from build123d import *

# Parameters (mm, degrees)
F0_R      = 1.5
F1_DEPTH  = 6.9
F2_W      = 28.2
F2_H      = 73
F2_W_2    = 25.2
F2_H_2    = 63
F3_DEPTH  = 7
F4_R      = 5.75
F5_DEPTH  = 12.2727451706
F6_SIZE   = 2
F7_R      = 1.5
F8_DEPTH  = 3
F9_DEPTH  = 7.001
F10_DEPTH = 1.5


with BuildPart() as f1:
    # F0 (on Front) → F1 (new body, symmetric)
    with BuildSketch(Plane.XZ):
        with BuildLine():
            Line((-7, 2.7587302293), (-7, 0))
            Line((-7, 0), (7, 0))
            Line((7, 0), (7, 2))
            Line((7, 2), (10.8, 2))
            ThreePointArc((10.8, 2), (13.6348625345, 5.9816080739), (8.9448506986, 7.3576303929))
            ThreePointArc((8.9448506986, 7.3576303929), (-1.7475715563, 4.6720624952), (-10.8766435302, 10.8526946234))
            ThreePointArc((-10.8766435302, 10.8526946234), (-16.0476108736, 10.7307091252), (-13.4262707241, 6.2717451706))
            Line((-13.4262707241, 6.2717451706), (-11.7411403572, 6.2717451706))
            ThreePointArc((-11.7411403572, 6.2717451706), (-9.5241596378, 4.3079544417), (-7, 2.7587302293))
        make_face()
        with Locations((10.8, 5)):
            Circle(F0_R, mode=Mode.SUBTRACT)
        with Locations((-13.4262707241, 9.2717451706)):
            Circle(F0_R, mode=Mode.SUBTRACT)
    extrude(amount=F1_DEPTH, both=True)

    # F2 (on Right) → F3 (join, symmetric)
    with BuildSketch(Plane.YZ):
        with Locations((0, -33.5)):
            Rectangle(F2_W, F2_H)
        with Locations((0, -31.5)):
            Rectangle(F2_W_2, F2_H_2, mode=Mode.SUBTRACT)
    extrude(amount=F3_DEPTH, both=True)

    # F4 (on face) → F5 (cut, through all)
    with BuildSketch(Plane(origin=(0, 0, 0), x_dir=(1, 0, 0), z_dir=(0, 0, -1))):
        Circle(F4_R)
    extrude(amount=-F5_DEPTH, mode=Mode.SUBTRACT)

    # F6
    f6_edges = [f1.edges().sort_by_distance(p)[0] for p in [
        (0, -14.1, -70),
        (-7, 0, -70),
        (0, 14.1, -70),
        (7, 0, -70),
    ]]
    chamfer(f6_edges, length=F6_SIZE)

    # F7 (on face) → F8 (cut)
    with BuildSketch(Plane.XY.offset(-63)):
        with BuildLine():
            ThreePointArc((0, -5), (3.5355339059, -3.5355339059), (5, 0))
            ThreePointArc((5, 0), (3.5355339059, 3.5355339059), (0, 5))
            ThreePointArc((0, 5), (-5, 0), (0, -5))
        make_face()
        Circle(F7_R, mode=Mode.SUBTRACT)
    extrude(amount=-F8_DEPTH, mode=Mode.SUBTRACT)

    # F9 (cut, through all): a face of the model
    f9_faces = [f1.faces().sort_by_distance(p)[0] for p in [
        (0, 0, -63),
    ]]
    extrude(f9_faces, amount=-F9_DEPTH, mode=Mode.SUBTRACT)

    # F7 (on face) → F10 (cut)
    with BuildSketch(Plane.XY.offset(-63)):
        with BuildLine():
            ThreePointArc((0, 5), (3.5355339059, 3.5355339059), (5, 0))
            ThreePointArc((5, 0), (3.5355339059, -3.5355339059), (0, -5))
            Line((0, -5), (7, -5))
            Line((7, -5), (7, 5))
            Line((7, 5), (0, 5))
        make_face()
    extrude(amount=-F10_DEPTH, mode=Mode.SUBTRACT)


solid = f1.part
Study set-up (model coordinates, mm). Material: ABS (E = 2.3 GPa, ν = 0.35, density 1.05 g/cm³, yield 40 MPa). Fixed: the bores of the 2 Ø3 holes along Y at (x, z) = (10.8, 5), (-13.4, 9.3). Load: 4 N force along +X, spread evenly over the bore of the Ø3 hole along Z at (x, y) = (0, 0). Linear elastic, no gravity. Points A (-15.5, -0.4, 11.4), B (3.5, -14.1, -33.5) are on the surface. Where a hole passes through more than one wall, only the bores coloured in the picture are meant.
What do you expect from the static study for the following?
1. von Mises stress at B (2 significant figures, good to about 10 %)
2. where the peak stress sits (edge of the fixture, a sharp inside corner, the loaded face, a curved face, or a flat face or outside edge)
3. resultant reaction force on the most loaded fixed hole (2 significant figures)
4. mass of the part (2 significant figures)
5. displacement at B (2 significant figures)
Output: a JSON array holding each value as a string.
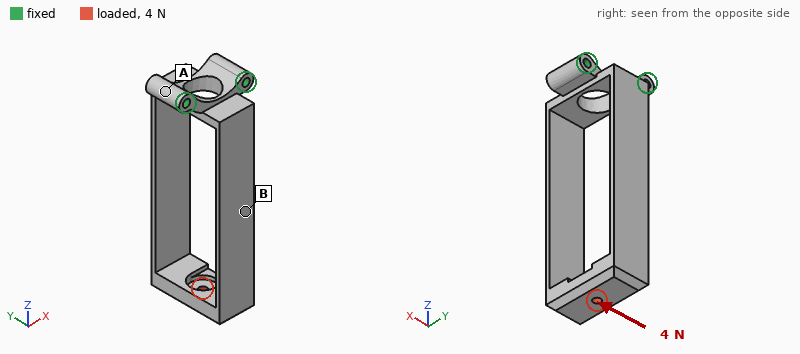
["0.81 MPa", "a flat face or outside edge", "19 N", "7.3 g", "0.39 mm"]
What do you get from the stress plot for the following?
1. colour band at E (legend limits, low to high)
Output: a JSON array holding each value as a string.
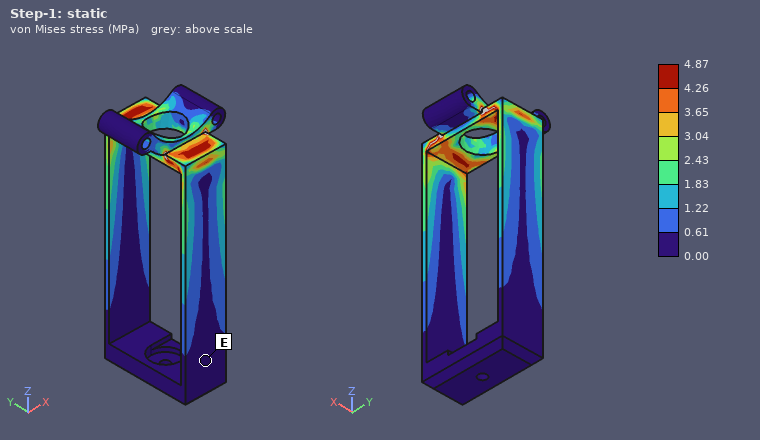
["0.00 to 0.61 MPa"]
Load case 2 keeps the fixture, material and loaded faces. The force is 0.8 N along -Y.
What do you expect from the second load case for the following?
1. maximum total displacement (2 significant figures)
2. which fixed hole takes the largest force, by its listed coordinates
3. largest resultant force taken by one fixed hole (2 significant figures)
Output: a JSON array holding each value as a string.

["1.1 mm", "(10.8, 5)", "0.62 N"]
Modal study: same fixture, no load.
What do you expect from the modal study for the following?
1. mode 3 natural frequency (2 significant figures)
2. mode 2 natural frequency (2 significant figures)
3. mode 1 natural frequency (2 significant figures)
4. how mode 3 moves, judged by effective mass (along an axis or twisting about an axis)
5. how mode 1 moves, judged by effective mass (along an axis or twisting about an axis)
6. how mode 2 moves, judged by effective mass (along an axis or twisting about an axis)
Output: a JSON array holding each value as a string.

["460 Hz", "200 Hz", "75 Hz", "twisting about Z", "along Y", "along X"]
